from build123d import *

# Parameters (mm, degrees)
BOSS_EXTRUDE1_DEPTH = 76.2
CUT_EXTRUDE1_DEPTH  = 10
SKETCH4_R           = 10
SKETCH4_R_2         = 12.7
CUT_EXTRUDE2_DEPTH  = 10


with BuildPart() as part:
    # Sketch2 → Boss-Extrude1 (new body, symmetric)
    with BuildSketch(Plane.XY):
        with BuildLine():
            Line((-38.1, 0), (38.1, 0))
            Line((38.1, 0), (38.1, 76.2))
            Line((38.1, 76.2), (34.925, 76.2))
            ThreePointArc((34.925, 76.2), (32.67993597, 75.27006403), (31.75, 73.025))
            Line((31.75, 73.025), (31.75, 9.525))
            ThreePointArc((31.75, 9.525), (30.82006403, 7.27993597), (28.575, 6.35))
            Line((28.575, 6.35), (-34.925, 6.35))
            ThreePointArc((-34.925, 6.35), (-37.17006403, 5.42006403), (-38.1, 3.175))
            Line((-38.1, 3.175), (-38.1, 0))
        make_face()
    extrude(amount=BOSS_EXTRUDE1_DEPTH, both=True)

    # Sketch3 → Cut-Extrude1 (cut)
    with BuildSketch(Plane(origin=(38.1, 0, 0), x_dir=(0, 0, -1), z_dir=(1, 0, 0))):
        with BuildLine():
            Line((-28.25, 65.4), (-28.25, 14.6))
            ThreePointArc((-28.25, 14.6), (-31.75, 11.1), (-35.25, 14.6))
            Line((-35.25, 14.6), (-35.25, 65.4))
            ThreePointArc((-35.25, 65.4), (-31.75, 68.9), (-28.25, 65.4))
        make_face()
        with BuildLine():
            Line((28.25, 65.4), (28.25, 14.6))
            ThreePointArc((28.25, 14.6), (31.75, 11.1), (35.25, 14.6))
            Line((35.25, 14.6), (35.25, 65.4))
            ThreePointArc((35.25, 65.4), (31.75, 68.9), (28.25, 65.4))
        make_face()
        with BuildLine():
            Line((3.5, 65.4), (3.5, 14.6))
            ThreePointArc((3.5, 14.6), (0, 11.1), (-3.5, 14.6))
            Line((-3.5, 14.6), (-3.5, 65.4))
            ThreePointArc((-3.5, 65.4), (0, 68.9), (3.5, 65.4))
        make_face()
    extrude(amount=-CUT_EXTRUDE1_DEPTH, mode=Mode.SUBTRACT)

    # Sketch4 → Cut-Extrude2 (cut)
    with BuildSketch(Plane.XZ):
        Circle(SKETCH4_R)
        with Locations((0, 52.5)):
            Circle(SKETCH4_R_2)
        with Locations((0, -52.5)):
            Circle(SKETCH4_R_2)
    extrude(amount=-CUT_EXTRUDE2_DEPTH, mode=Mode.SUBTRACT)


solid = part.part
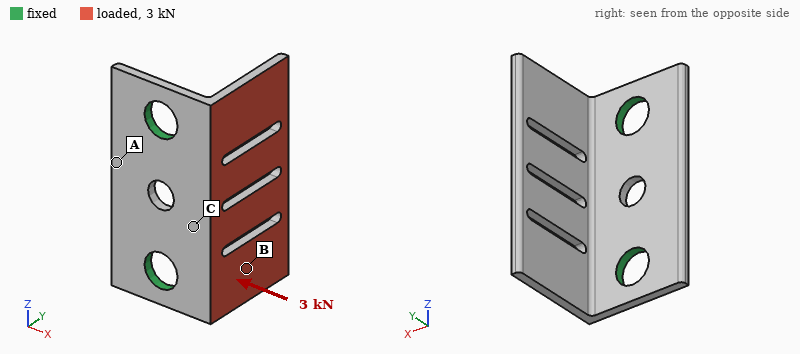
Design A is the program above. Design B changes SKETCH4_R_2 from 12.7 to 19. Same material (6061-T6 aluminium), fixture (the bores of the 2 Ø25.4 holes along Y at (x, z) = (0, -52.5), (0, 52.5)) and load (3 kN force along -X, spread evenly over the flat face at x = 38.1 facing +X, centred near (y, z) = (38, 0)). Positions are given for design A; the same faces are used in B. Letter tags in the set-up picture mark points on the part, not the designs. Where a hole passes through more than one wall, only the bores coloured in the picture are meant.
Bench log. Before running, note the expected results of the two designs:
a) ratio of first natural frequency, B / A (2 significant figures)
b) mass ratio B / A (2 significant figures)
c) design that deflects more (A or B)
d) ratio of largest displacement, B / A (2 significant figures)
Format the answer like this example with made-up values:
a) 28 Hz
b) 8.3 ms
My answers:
a) 1.1
b) 0.94
c) A
d) 0.82
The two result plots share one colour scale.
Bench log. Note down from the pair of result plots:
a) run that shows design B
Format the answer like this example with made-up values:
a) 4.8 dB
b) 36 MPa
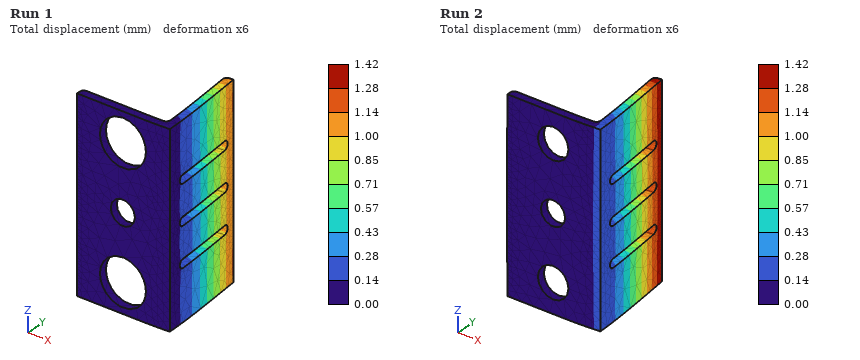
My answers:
a) Run 1
